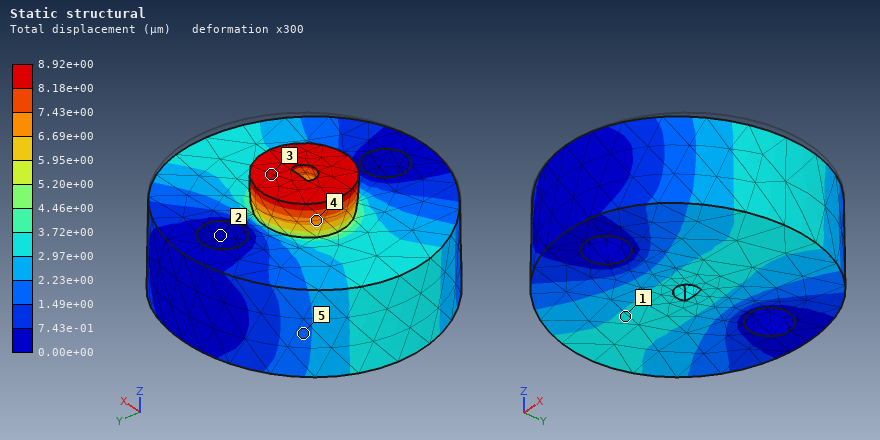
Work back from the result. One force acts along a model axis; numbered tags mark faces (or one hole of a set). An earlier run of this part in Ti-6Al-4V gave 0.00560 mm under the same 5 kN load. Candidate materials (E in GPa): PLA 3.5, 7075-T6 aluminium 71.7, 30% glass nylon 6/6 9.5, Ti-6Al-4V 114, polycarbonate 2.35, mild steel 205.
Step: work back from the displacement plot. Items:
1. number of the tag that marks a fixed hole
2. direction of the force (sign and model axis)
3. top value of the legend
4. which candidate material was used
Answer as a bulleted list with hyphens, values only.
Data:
- 2
- -Z
- 8.92e+00 µm
- 7075-T6 aluminium
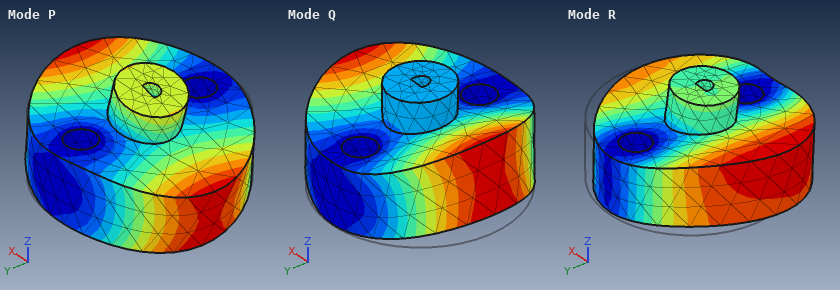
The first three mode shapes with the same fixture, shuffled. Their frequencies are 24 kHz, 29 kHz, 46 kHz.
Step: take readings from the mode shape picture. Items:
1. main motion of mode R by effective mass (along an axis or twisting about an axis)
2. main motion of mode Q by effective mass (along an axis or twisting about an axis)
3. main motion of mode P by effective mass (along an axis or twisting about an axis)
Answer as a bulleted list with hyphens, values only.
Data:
- along Y
- along Z
- twisting about Y
